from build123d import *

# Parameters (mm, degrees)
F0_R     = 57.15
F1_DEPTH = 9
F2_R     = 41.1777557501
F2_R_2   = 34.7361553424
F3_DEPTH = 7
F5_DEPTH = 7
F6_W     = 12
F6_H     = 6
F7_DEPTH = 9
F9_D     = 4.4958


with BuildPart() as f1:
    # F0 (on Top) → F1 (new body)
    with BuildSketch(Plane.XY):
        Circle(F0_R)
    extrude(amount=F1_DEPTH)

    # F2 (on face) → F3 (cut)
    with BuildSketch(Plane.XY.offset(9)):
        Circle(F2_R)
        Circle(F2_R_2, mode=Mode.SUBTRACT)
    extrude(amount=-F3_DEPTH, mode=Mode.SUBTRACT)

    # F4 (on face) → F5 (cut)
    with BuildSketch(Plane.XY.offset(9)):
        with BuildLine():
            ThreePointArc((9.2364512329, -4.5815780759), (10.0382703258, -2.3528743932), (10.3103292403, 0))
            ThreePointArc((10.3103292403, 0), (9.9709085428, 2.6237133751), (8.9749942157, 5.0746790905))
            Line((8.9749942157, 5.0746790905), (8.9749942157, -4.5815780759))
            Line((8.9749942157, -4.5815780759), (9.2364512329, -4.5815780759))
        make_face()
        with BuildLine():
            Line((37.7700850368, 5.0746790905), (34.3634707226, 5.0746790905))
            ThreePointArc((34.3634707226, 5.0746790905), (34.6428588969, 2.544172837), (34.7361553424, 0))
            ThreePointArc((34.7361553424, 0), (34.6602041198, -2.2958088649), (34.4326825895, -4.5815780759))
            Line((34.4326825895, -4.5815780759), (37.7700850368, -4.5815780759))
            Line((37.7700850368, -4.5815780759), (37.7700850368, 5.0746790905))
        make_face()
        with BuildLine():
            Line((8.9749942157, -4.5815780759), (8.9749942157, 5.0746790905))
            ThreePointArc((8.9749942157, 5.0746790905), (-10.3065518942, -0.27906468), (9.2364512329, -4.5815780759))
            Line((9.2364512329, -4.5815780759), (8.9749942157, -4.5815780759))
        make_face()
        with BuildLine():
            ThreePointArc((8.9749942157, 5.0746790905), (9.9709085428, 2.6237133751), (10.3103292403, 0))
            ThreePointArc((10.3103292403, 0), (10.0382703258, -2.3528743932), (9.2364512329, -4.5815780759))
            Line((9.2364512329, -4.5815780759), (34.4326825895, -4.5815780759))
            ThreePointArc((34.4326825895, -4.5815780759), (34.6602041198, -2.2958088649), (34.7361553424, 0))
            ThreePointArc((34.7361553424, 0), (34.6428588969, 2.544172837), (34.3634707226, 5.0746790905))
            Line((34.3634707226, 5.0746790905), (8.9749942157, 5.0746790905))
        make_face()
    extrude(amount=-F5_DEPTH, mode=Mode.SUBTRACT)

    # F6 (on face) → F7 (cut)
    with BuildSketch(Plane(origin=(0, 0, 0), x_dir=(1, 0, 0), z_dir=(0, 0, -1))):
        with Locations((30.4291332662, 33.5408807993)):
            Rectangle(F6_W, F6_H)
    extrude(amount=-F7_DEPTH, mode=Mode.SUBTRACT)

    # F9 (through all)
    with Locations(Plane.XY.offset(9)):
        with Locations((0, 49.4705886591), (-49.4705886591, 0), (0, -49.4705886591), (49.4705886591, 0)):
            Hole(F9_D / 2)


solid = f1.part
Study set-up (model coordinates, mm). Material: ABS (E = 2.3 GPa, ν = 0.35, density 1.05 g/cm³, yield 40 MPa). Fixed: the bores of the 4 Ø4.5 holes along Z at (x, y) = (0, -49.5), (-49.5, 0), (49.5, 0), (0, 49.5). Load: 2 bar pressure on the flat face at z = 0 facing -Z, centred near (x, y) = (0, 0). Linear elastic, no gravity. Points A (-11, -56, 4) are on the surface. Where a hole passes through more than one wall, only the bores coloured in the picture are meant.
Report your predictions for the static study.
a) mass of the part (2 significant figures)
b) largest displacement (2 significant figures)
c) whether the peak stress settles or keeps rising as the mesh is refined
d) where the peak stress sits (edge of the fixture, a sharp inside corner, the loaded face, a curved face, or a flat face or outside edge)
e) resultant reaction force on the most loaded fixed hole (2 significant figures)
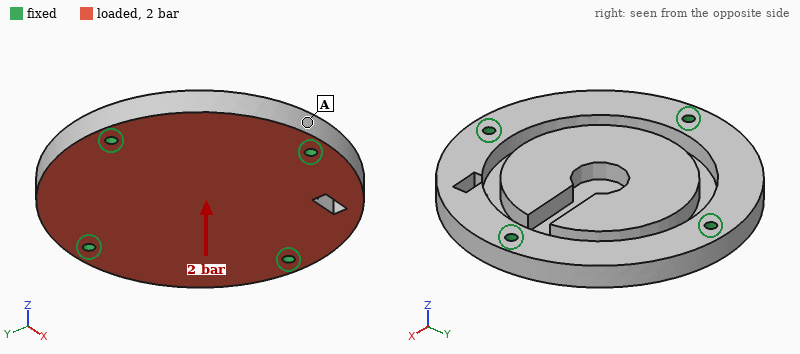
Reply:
80 g
0.63 mm
keeps rising
edge of the fixture
530 N
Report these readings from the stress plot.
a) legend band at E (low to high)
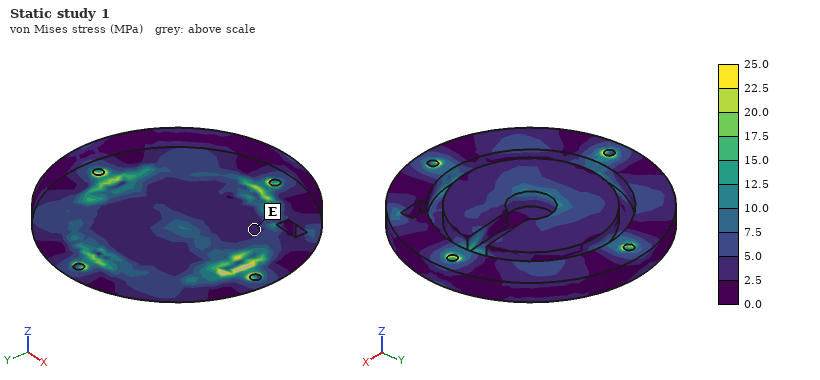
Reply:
2.5 to 5.0 MPa
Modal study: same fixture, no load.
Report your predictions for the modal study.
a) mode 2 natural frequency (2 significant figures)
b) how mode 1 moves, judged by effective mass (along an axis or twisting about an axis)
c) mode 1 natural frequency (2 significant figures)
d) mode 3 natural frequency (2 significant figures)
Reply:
1900 Hz
along Z
1300 Hz
1900 Hz
